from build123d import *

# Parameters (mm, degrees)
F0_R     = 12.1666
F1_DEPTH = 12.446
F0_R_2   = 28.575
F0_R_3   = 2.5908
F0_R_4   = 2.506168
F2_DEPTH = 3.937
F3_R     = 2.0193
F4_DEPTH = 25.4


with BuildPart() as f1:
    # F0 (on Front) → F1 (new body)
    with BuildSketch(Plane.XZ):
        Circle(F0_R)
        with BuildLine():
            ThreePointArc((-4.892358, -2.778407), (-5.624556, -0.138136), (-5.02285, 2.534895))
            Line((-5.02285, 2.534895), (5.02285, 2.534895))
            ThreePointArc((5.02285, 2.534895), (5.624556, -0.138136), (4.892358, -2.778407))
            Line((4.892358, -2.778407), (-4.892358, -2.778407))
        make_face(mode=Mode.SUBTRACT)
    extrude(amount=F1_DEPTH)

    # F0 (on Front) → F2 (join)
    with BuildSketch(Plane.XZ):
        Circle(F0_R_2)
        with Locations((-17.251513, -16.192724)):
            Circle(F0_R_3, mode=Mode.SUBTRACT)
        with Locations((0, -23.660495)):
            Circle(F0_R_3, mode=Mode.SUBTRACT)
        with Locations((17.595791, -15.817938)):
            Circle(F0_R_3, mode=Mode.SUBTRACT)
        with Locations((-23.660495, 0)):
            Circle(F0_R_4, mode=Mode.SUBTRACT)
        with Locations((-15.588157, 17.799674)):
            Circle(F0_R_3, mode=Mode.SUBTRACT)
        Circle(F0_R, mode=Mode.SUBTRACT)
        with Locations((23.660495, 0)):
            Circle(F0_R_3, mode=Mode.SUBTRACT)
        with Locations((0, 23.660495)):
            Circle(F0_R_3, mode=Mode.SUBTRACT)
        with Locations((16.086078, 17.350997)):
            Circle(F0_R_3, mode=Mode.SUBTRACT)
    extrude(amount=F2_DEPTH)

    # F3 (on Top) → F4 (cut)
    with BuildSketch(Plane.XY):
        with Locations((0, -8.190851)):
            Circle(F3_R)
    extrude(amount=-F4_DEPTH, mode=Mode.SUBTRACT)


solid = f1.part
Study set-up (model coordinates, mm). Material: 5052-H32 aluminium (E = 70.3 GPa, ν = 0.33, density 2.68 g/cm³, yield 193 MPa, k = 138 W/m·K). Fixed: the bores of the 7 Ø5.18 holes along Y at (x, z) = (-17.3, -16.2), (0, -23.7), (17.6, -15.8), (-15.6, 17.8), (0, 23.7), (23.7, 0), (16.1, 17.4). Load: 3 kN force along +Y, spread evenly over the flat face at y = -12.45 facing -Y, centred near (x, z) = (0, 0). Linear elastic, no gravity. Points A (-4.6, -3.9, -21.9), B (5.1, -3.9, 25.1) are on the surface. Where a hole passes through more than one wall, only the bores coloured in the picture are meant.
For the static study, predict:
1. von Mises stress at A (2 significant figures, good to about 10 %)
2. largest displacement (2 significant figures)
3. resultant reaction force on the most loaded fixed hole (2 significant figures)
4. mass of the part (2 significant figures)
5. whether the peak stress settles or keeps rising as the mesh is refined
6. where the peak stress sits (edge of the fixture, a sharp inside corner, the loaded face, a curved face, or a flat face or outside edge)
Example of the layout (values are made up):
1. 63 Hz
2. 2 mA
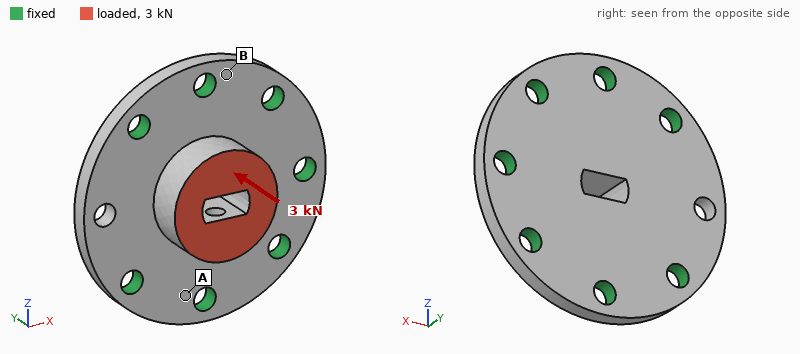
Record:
1. 22 MPa
2. 22 µm
3. 630 N
4. 34 g
5. keeps rising
6. edge of the fixture
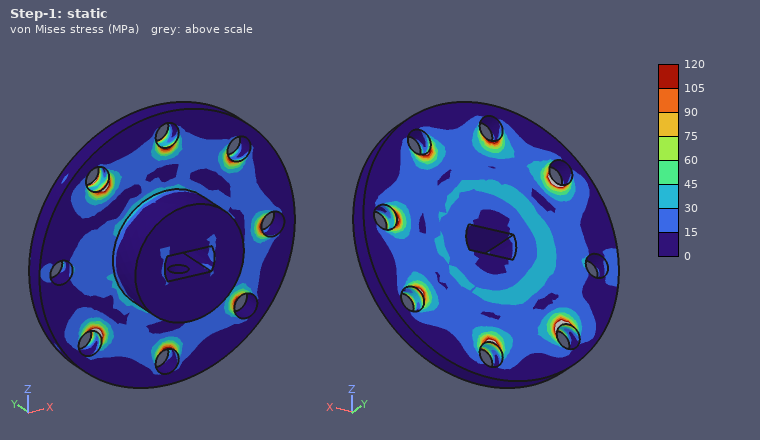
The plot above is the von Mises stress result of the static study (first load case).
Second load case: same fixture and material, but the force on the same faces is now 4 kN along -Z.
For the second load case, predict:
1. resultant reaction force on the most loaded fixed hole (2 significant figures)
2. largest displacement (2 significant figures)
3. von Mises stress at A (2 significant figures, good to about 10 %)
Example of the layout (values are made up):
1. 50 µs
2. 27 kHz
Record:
1. 1.0 kN
2. 32 µm
3. 16 MPa
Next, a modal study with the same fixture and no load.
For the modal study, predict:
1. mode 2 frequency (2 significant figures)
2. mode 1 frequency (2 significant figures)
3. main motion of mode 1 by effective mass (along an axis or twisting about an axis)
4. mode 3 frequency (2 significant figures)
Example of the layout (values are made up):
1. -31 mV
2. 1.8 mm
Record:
1. 18 kHz
2. 15 kHz
3. along Y
4. 23 kHz
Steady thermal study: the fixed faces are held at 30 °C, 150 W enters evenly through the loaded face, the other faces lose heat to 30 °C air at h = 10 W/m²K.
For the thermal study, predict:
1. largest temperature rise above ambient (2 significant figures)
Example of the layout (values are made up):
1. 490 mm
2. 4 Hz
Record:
1. 69 K
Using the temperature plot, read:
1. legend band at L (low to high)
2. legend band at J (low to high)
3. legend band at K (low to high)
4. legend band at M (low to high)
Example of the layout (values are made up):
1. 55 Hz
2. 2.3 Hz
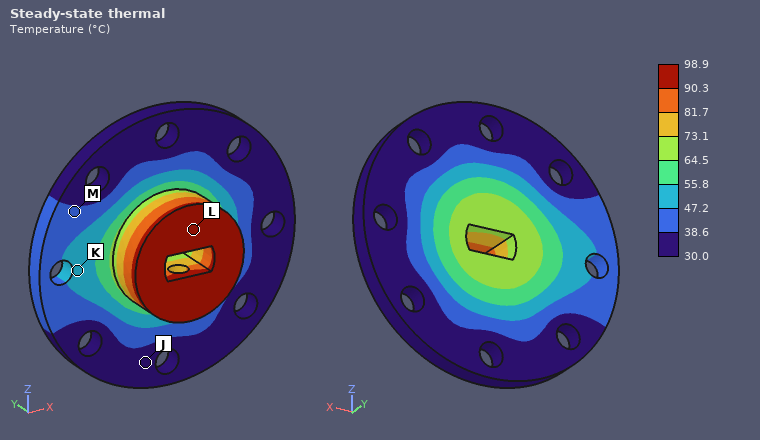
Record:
1. 90.3 to 98.9 °C
2. 30.0 to 38.6 °C
3. 47.2 to 55.8 °C
4. 38.6 to 47.2 °C
